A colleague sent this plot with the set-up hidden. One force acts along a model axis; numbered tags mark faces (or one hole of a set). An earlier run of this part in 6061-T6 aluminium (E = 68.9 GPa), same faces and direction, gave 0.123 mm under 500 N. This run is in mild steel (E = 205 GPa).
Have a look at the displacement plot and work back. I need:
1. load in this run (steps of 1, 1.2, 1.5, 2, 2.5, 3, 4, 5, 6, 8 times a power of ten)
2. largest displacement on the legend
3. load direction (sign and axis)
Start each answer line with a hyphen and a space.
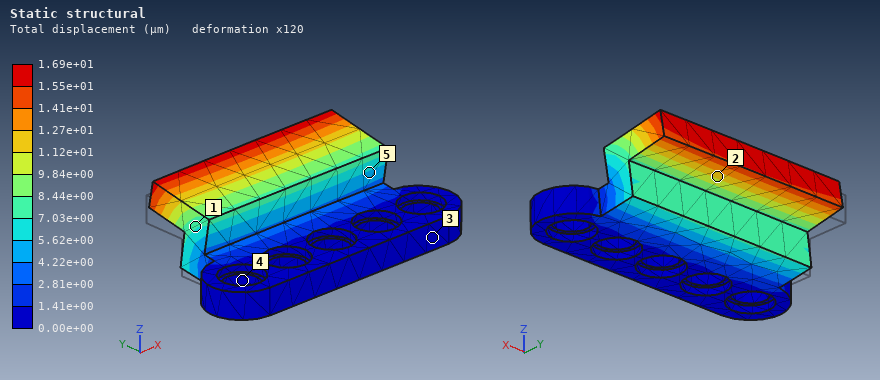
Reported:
- 200 N
- 1.69e+01 µm
- +Z
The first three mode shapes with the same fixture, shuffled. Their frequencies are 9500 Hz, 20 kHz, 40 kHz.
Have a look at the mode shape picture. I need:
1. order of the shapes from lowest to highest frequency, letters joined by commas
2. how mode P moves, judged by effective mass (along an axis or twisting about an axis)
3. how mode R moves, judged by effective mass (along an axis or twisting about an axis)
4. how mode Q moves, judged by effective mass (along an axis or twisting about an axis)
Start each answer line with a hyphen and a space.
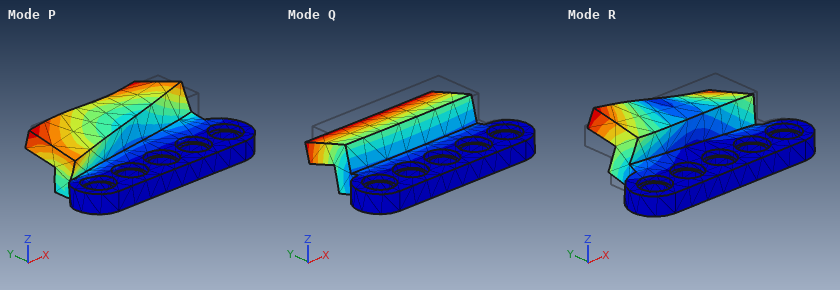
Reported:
- Q, R, P
- along X
- twisting about Y
- along Z
